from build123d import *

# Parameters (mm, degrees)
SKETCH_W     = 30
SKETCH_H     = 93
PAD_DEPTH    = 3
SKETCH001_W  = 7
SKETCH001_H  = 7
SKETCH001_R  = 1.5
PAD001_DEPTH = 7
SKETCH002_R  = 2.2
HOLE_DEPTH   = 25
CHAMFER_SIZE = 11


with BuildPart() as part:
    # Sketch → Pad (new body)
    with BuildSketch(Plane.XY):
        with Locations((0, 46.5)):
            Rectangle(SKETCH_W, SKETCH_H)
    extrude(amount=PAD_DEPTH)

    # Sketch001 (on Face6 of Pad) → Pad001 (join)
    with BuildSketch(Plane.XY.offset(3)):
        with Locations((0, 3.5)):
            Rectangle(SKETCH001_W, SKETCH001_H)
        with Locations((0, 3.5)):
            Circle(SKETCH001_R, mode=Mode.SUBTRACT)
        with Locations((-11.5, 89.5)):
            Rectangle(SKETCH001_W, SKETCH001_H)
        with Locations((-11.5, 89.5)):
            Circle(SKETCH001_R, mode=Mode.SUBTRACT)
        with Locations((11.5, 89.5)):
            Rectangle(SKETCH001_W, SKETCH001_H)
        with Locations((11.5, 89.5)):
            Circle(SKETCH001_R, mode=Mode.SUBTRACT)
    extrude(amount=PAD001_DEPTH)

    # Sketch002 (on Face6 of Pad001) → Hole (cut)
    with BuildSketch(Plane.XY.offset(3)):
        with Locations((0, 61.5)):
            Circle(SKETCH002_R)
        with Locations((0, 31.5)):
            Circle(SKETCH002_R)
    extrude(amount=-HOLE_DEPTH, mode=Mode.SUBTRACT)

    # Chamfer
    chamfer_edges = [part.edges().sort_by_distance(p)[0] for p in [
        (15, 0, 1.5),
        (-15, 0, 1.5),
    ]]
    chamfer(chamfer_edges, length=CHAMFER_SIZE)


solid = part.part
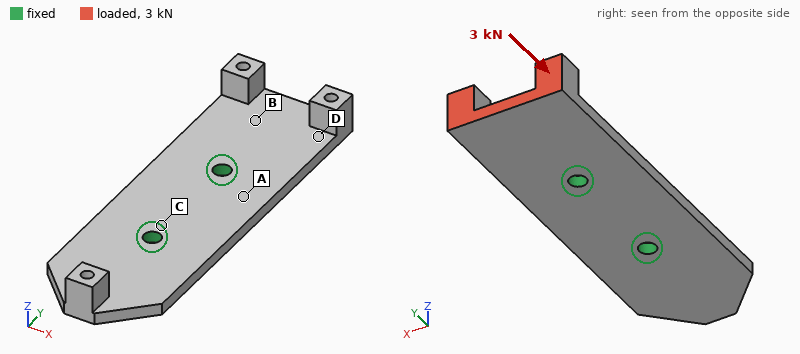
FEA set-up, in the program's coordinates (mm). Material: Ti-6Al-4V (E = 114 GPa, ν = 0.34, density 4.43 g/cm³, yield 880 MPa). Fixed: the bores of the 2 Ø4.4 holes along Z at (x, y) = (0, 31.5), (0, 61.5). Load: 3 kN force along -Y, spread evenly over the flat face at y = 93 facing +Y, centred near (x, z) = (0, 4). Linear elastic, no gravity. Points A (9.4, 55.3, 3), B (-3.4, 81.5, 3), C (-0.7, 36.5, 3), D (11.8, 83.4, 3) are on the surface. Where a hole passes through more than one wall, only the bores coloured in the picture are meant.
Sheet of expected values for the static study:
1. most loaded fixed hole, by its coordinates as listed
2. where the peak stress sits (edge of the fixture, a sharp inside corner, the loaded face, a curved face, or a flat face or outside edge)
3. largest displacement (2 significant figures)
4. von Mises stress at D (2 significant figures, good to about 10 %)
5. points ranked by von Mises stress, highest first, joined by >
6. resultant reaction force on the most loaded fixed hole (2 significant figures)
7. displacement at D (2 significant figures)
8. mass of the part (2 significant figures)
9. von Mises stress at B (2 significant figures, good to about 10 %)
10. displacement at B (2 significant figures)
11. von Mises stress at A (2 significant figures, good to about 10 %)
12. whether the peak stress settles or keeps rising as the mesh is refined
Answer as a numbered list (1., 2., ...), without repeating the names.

1. (0, 61.5)
2. edge of the fixture
3. 0.54 mm
4. 230 MPa
5. D > B > A > C
6. 2.4 kN
7. 0.24 mm
8. 39 g
9. 180 MPa
10. 0.21 mm
11. 40 MPa
12. keeps rising
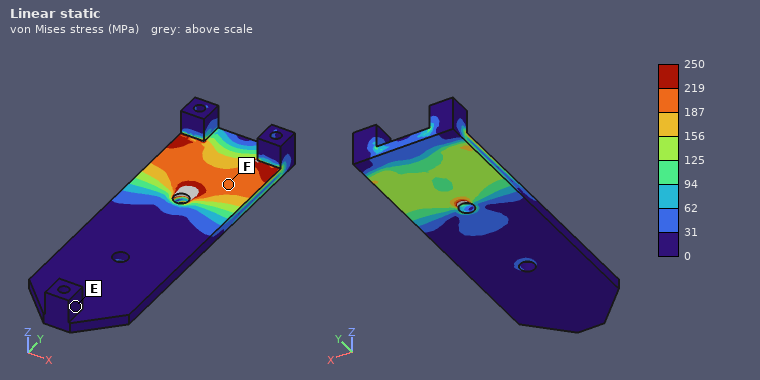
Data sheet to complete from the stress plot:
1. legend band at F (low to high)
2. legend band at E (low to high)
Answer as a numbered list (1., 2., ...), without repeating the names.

1. 187 to 219 MPa
2. 0 to 31 MPa
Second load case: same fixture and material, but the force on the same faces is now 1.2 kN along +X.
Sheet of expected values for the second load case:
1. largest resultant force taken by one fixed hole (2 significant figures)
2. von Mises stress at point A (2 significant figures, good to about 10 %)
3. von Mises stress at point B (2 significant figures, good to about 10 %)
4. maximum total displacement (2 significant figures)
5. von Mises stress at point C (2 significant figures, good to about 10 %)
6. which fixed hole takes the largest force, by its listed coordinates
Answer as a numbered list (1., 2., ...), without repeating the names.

1. 2.2 kN
2. 25 MPa
3. 79 MPa
4. 0.16 mm
5. 22 MPa
6. (0, 61.5)
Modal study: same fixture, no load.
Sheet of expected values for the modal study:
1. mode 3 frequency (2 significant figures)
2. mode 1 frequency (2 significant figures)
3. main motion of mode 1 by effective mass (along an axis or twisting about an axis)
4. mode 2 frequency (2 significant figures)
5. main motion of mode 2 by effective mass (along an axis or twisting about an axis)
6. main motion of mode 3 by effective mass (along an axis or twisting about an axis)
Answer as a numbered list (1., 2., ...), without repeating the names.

1. 3500 Hz
2. 1900 Hz
3. along Z
4. 2500 Hz
5. along Z
6. twisting about Y
